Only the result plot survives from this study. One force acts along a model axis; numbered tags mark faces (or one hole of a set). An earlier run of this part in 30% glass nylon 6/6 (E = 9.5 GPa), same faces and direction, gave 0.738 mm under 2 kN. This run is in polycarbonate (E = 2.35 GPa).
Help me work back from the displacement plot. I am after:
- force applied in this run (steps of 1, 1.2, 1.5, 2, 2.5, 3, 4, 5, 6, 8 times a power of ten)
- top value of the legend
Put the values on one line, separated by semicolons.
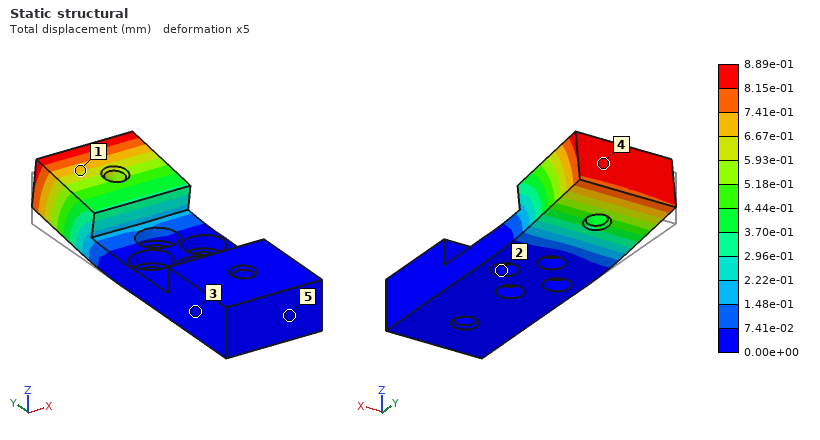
600 N; 8.89e-01 mm
